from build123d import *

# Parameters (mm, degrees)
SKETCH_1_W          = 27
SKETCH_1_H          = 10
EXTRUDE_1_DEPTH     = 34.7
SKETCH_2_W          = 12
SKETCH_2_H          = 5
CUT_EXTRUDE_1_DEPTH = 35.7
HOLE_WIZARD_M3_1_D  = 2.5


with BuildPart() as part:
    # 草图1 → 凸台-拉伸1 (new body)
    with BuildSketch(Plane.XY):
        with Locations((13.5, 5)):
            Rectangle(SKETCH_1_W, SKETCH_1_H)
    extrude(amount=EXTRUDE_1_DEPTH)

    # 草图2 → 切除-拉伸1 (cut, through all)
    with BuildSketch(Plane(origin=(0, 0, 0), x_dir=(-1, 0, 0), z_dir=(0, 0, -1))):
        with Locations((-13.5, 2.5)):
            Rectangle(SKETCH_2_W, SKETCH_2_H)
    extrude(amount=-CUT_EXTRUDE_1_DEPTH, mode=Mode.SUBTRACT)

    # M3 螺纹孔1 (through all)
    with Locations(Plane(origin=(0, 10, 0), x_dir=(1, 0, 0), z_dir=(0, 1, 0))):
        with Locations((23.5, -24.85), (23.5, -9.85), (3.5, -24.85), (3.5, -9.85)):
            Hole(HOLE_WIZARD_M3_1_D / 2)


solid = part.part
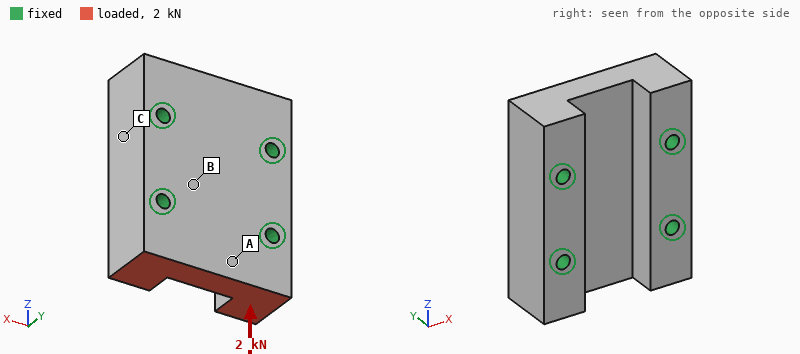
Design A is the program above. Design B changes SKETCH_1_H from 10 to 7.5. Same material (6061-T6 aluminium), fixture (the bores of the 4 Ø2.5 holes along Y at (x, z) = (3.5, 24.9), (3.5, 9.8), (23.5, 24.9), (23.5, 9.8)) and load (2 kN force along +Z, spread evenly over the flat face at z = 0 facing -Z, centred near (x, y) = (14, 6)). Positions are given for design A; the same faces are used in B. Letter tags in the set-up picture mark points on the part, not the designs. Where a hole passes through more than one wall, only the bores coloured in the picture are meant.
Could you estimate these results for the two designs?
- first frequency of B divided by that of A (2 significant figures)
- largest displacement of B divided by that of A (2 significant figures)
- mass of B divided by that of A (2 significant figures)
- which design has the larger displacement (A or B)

0.88
1.3
0.75
B
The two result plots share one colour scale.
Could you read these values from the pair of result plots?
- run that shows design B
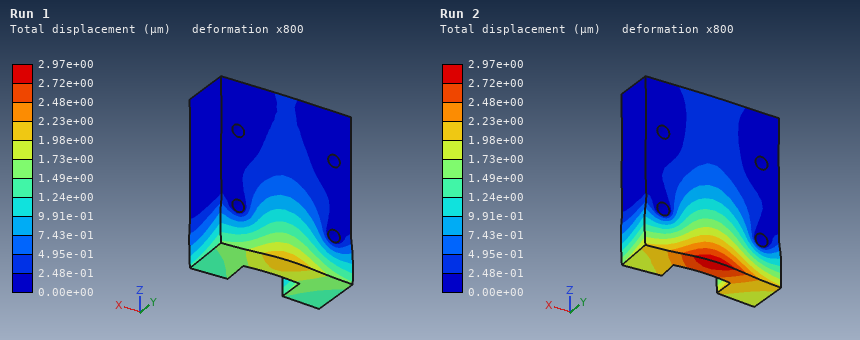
Run 2
